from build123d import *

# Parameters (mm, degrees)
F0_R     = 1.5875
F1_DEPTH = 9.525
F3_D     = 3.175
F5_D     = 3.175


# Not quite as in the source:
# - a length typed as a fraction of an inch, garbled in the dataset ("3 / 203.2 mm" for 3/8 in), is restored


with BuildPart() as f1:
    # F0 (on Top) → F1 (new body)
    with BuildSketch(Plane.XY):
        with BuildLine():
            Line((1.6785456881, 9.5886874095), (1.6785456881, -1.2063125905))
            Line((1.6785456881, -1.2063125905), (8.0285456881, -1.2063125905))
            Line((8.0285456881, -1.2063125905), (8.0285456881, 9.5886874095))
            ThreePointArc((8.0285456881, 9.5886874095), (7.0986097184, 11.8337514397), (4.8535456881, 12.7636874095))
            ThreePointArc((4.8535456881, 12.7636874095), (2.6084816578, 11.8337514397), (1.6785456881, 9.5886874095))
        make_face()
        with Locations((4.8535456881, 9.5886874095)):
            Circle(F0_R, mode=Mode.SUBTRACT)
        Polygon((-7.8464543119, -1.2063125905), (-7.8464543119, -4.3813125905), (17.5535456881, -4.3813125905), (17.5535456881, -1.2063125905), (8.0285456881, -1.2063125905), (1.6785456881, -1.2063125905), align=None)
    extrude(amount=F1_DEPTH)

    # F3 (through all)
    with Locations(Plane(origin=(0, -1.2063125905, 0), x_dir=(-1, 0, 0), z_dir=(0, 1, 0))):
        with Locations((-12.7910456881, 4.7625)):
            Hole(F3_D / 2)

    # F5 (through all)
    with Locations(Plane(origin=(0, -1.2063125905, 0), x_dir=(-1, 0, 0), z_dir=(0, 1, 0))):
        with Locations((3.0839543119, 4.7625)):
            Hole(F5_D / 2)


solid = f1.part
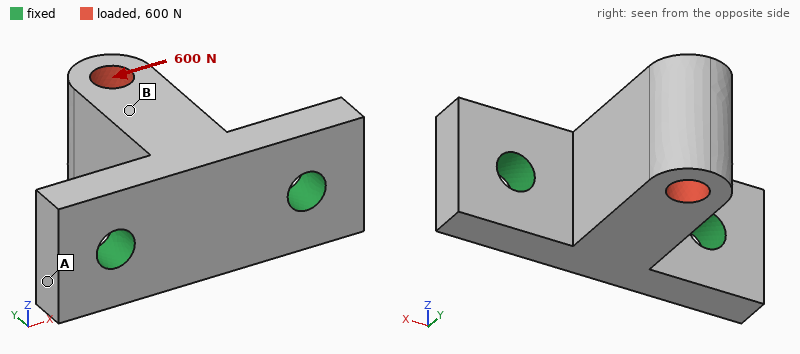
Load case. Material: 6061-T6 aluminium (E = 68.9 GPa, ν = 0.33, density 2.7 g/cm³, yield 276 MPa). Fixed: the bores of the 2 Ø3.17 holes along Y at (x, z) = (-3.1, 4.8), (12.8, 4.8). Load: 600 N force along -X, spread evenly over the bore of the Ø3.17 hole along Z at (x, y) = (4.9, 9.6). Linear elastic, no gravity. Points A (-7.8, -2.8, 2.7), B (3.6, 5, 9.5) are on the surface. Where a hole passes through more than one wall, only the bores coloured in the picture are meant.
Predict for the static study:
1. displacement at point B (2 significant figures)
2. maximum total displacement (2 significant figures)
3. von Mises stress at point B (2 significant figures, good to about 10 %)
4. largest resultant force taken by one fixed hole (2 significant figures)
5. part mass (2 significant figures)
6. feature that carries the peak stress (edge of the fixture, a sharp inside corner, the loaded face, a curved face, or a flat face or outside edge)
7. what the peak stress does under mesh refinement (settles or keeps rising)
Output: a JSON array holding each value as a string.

["26 µm", "66 µm", "30 MPa", "730 N", "3.9 g", "edge of the fixture", "keeps rising"]
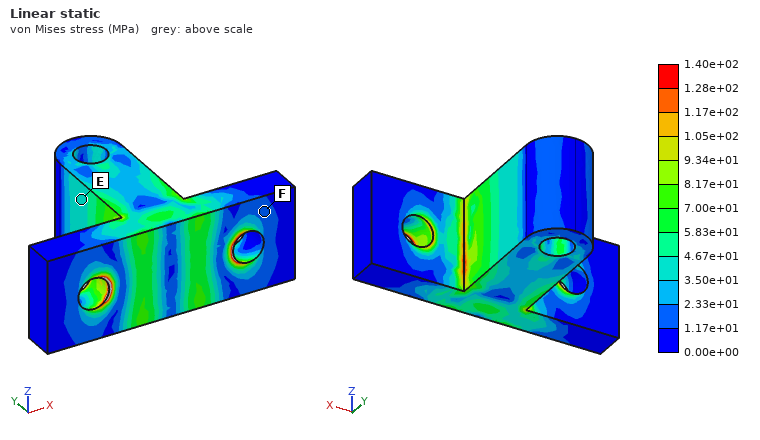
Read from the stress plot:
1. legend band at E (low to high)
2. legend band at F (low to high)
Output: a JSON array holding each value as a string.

["3.50e+01 to 4.67e+01 MPa", "1.17e+01 to 2.33e+01 MPa"]
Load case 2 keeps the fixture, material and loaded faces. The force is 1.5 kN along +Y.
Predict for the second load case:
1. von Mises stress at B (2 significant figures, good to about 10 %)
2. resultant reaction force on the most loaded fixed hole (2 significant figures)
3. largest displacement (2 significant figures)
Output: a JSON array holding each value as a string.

["23 MPa", "780 N", "18 µm"]
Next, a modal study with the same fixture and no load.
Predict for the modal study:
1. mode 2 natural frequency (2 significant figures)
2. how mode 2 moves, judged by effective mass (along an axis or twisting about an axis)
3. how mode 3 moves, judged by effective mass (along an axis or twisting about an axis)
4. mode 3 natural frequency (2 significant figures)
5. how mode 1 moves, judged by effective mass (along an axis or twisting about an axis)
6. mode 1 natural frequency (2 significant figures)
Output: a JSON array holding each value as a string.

["18 kHz", "along X", "along Y", "34 kHz", "along Z", "12 kHz"]
